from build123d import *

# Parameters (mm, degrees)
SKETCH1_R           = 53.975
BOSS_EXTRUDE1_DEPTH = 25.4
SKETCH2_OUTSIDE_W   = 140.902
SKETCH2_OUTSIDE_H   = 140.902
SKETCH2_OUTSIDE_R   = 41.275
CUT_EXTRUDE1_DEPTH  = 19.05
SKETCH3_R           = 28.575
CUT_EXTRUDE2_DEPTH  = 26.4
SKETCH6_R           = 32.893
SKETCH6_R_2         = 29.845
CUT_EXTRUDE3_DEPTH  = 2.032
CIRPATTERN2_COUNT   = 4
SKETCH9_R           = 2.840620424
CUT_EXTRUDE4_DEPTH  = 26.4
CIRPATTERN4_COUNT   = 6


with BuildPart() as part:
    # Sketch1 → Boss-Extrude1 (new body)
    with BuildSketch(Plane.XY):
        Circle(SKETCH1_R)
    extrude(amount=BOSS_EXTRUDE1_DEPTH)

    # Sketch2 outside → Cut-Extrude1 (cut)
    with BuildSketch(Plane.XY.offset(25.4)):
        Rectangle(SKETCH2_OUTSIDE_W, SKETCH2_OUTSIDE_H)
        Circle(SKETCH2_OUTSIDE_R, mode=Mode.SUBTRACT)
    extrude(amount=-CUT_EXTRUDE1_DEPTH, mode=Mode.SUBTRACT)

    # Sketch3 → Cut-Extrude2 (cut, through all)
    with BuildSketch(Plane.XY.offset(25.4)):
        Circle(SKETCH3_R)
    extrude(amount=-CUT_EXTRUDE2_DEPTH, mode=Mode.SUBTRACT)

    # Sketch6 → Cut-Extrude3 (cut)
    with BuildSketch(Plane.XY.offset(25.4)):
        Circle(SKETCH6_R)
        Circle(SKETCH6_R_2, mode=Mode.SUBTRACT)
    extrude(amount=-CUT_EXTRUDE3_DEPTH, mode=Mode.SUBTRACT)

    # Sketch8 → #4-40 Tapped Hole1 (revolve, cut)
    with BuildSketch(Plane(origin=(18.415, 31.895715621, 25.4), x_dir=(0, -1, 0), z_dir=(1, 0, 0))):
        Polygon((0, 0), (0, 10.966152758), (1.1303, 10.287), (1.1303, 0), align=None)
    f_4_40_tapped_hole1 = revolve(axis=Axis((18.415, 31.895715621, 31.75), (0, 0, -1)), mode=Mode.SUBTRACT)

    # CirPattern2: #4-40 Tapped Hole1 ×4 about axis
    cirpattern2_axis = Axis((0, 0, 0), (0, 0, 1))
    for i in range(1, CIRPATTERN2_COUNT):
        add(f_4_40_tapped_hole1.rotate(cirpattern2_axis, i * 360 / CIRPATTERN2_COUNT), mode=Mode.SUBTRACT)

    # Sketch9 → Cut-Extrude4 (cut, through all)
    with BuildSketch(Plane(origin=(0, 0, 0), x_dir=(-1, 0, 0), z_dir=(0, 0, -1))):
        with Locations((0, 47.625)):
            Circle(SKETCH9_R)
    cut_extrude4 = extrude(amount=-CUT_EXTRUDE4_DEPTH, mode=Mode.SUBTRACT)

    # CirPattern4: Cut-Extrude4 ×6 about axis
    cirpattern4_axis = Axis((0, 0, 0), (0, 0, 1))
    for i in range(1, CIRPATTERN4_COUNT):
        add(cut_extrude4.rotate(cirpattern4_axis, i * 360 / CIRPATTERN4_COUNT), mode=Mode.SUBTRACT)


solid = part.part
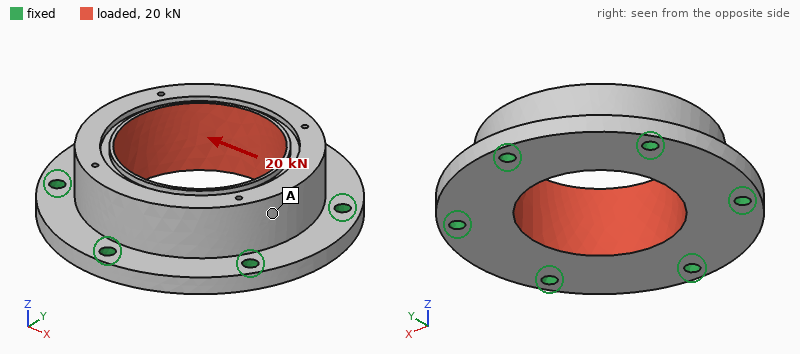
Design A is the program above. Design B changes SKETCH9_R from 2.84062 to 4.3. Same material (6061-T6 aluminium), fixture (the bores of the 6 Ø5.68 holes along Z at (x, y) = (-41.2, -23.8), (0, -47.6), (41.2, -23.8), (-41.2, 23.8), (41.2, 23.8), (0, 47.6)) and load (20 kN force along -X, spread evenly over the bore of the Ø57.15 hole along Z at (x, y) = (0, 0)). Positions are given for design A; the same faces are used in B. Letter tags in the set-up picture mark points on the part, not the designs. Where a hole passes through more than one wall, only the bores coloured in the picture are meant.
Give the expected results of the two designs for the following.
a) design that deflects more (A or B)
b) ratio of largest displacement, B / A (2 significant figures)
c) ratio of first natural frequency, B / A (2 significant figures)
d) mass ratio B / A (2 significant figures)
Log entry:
A
0.92
1.2
0.99
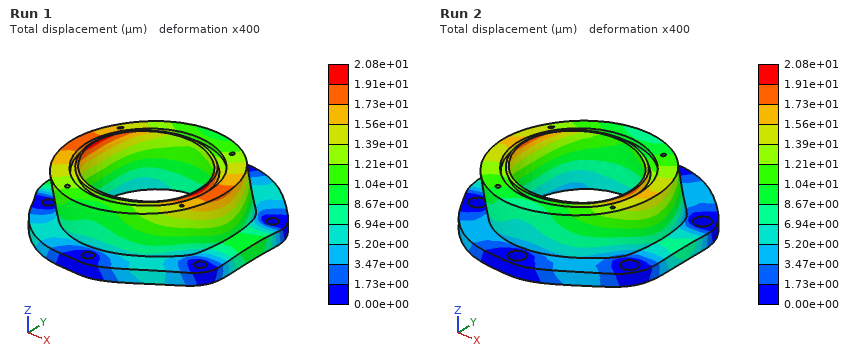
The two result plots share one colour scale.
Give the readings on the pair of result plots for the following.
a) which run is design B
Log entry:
Run 2
